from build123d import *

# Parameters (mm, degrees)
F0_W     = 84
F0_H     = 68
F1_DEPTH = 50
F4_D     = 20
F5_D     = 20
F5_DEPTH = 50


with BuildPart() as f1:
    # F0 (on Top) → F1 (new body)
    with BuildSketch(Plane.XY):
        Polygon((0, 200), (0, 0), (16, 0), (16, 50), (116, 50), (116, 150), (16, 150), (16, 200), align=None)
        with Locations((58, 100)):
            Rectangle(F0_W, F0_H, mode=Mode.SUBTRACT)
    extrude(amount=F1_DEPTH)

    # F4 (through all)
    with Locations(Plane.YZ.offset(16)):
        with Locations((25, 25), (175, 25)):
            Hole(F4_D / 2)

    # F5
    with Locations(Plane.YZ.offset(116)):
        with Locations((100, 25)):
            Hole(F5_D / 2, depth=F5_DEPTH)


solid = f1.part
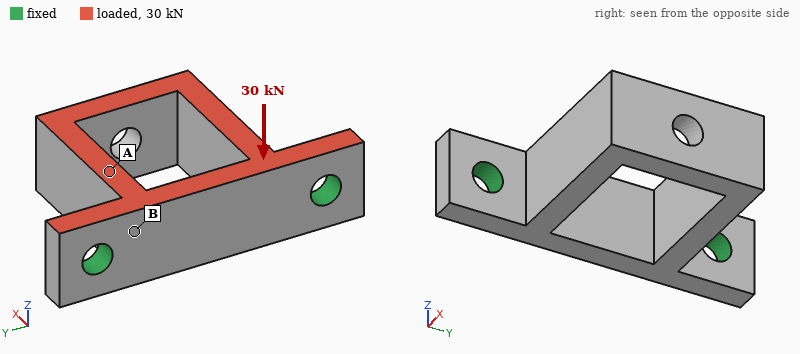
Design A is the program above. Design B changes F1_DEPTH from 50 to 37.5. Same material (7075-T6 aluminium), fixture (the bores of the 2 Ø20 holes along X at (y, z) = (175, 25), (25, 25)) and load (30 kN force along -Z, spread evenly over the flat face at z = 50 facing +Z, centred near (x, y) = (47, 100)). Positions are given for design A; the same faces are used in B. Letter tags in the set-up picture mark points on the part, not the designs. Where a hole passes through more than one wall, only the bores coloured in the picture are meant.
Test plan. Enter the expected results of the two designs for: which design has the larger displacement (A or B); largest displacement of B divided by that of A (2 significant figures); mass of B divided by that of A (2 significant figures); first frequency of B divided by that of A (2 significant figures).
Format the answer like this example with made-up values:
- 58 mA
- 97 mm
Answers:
- B
- 1.7
- 0.74
- 0.90
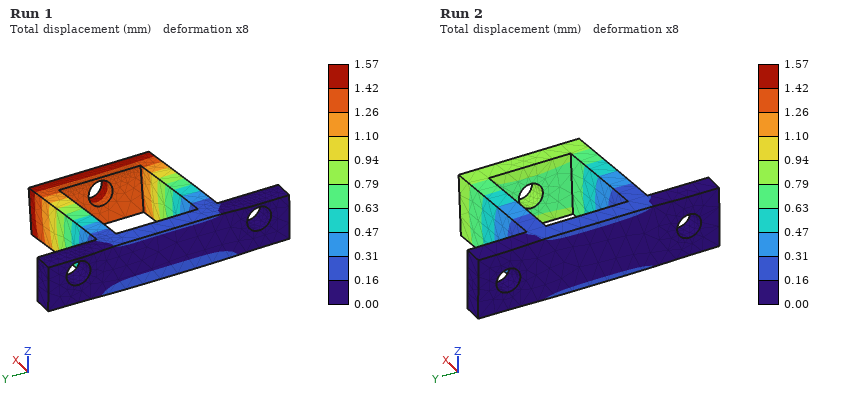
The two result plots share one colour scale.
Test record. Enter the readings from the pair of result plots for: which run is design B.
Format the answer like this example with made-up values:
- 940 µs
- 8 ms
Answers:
- Run 1
